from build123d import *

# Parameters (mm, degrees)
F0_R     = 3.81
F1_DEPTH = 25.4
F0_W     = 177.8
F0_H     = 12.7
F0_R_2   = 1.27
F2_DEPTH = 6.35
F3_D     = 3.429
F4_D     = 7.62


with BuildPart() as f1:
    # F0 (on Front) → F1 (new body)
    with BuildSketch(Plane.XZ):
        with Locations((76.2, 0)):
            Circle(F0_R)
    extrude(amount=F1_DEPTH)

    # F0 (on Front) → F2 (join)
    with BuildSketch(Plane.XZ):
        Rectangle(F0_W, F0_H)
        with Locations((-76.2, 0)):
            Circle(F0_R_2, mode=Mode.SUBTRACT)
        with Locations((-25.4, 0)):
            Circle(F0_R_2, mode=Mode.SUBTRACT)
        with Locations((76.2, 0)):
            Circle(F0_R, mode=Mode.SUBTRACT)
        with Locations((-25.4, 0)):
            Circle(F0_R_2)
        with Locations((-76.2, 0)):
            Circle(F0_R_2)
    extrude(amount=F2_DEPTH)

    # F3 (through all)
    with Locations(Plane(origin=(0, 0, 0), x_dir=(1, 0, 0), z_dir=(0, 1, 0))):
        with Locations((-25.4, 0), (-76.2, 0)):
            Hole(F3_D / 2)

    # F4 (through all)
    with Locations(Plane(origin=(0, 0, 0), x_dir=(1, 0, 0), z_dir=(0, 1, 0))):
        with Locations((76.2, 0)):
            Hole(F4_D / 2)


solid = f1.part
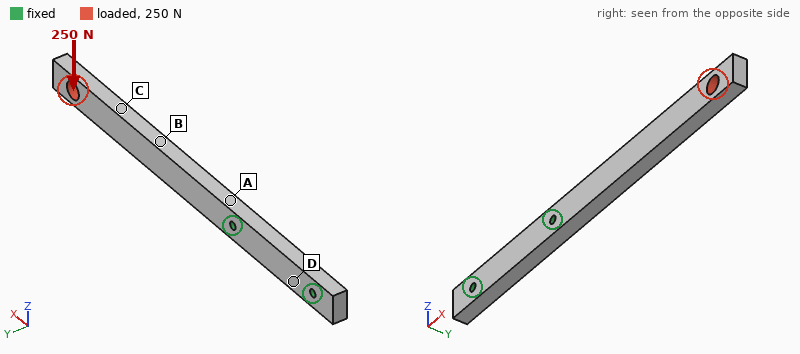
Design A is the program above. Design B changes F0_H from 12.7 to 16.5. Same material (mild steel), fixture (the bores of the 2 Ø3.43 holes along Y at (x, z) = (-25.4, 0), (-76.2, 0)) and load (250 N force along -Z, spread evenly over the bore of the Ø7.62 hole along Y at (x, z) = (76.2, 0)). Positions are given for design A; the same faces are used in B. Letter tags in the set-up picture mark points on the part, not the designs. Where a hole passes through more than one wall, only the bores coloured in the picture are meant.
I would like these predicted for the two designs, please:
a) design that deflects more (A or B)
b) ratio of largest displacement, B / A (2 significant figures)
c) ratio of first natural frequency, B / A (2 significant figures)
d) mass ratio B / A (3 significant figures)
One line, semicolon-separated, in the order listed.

A; 0.50; 0.98; 1.31
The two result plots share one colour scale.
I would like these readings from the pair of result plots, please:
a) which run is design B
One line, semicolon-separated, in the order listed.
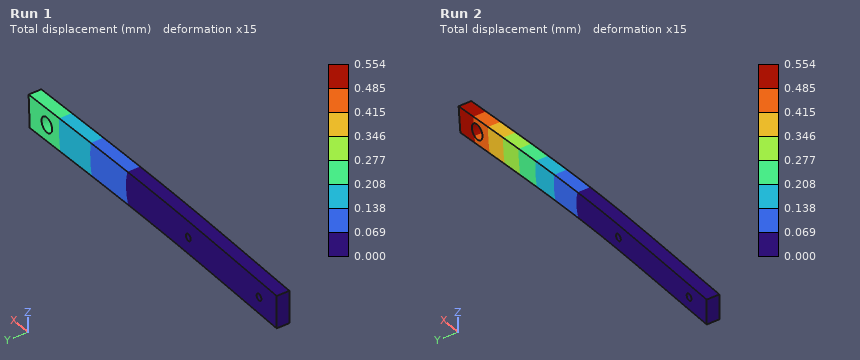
Run 1
